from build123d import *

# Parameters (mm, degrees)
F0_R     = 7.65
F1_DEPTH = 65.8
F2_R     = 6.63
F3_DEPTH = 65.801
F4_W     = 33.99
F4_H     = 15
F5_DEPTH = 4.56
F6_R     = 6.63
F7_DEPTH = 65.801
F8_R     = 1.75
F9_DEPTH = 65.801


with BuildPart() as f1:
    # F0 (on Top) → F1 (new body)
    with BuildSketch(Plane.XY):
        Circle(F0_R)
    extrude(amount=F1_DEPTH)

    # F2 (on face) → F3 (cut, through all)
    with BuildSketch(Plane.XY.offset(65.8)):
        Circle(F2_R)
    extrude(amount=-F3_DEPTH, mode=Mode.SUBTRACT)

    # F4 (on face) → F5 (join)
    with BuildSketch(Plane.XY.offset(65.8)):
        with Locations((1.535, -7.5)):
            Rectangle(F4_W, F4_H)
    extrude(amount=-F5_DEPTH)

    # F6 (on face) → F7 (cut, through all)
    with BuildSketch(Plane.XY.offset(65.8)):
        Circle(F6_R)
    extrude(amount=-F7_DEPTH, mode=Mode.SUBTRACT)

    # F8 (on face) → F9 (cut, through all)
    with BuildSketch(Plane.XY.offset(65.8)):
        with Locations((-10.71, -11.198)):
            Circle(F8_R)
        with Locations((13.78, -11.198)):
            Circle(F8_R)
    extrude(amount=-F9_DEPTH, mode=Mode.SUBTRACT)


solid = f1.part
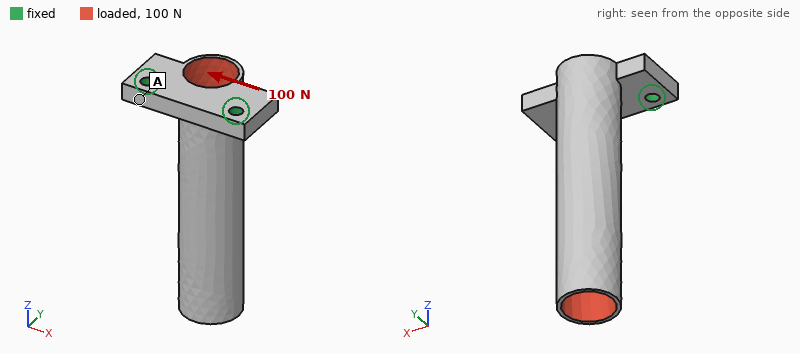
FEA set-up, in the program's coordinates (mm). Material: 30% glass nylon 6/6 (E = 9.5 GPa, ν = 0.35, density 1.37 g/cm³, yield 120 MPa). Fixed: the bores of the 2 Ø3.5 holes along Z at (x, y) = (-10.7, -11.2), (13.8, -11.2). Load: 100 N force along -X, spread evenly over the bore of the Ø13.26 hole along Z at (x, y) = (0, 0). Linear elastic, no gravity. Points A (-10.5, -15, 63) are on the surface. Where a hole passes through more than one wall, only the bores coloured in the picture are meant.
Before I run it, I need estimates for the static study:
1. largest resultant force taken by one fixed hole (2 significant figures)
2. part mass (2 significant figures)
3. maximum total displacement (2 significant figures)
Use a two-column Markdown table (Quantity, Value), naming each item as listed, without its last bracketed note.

| Quantity | Value |
|---|---|
| largest resultant force taken by one fixed hole | 170 N |
| part mass | 6.6 g |
| maximum total displacement | 0.82 mm |
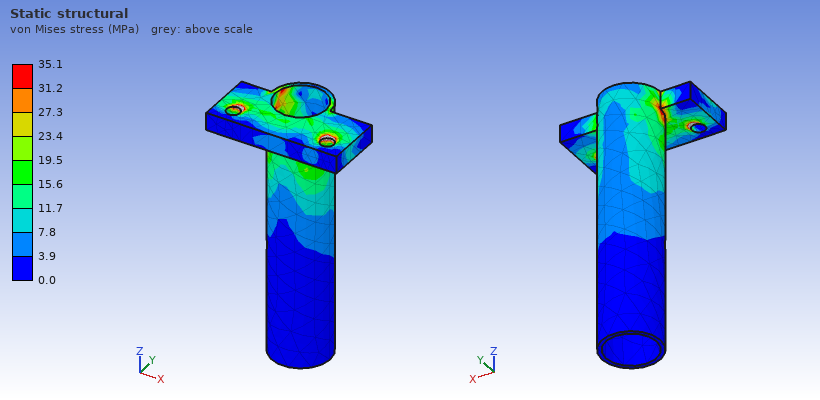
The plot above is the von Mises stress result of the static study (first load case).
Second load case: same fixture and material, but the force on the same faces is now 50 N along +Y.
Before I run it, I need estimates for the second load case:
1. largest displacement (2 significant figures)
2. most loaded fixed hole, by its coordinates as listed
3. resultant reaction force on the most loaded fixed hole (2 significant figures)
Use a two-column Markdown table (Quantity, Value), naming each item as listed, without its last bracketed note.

| Quantity | Value |
|---|---|
| largest displacement | 0.89 mm |
| most loaded fixed hole, by its coordinates as listed | (-10.7, -11.2) |
| resultant reaction force on the most loaded fixed hole | 34 N |
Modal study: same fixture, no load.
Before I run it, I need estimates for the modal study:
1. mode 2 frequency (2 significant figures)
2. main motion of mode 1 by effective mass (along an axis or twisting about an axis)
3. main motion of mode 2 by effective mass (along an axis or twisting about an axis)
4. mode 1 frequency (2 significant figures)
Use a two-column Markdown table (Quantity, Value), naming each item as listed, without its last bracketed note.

| Quantity | Value |
|---|---|
| mode 2 frequency | 1100 Hz |
| main motion of mode 1 by effective mass | along Y |
| main motion of mode 2 by effective mass | along X |
| mode 1 frequency | 710 Hz |
